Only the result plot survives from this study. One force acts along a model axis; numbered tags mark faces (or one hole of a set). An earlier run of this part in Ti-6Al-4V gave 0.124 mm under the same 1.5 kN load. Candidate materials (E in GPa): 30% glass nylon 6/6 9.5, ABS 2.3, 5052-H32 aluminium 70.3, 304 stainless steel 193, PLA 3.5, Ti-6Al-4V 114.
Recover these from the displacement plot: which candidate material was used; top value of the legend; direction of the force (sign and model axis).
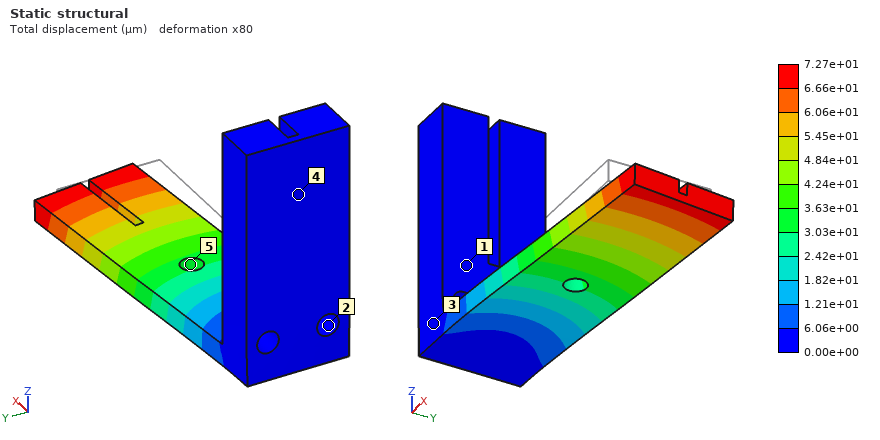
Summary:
304 stainless steel
7.27e+01 µm
+Y
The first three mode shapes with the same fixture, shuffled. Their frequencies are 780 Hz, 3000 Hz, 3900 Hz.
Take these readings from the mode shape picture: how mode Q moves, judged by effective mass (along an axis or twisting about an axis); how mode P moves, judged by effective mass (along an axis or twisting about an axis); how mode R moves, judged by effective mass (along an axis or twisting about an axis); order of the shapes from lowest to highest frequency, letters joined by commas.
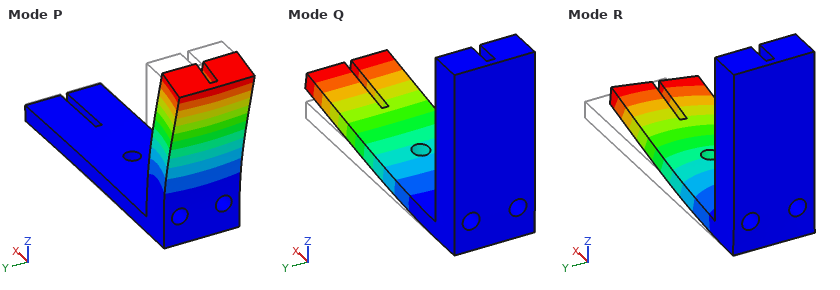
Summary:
along Z
along X
along Y
Q, R, P
